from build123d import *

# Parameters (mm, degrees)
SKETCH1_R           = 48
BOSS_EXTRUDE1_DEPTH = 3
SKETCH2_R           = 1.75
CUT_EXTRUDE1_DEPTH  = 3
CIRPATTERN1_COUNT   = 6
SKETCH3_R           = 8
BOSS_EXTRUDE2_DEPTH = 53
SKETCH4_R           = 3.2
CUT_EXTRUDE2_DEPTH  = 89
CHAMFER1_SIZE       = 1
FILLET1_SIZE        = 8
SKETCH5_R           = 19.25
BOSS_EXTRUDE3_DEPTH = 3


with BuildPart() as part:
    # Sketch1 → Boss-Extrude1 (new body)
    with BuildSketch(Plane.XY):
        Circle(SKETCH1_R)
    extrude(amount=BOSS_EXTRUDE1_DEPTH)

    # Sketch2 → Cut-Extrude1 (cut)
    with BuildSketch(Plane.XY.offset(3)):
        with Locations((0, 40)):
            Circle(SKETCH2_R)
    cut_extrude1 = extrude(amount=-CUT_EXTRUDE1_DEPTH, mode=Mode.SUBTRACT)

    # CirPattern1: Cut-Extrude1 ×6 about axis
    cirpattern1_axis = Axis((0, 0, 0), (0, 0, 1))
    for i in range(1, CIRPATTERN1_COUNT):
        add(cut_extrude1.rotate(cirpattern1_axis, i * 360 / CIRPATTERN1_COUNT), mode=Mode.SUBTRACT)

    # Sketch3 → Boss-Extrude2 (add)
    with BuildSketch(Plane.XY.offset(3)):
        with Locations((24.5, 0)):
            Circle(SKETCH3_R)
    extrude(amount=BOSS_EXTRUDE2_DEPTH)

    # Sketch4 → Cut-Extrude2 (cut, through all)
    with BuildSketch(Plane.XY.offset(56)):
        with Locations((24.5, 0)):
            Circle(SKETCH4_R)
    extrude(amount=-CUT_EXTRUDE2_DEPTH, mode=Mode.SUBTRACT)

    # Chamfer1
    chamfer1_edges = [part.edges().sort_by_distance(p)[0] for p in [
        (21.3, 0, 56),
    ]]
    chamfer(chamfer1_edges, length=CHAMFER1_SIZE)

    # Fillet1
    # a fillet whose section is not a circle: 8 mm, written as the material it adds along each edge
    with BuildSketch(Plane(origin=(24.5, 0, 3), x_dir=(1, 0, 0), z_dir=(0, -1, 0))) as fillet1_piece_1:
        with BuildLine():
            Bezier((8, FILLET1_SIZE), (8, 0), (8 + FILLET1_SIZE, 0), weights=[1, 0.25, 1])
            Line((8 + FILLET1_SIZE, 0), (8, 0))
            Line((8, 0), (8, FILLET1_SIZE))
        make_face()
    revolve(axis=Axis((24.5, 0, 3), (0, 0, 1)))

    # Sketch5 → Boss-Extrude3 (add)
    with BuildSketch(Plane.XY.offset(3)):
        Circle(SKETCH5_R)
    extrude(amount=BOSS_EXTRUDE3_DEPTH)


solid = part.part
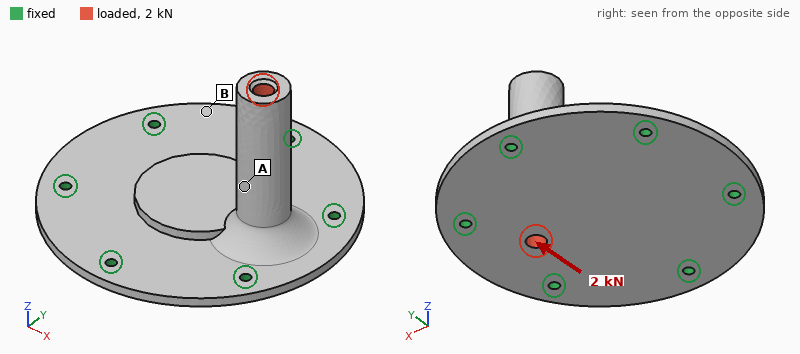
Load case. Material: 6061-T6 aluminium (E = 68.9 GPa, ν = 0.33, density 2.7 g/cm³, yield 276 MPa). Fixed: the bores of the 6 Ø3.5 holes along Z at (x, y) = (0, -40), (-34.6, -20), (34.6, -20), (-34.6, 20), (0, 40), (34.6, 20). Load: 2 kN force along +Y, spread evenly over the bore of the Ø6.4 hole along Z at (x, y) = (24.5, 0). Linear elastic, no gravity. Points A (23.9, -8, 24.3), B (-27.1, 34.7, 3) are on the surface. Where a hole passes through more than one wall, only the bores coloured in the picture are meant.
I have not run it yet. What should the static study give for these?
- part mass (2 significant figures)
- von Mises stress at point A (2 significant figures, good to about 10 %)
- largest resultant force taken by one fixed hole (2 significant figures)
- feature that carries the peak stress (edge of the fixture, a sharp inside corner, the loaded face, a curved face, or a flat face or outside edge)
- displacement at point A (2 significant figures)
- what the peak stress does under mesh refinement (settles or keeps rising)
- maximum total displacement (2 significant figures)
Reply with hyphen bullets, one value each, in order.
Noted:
- 94 g
- 43 MPa
- 1.4 kN
- edge of the fixture
- 0.12 mm
- keeps rising
- 0.32 mm
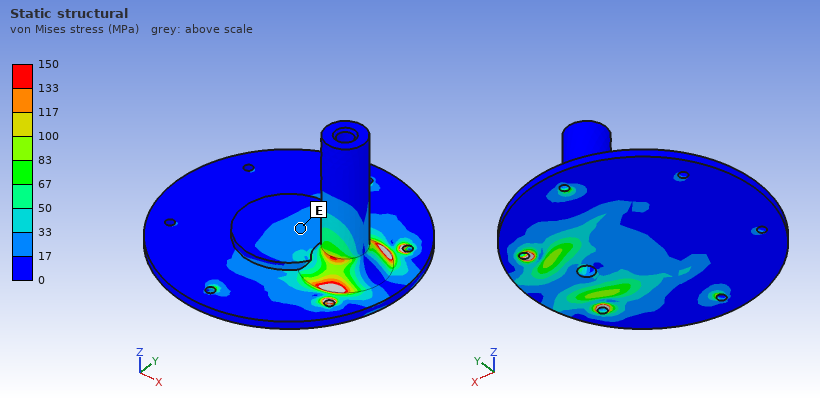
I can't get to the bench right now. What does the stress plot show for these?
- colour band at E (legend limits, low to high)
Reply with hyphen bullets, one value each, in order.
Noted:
- 17 to 33 MPa
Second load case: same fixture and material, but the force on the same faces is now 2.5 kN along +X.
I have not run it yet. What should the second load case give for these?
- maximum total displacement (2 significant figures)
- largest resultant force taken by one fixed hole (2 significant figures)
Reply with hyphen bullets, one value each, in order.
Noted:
- 0.60 mm
- 950 N
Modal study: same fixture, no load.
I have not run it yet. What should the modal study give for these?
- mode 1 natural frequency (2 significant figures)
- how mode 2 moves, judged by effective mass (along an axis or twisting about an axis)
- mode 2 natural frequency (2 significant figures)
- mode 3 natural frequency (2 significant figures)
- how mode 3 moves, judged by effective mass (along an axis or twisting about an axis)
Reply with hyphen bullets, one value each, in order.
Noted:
- 2300 Hz
- along Y
- 3000 Hz
- 4800 Hz
- along Z
